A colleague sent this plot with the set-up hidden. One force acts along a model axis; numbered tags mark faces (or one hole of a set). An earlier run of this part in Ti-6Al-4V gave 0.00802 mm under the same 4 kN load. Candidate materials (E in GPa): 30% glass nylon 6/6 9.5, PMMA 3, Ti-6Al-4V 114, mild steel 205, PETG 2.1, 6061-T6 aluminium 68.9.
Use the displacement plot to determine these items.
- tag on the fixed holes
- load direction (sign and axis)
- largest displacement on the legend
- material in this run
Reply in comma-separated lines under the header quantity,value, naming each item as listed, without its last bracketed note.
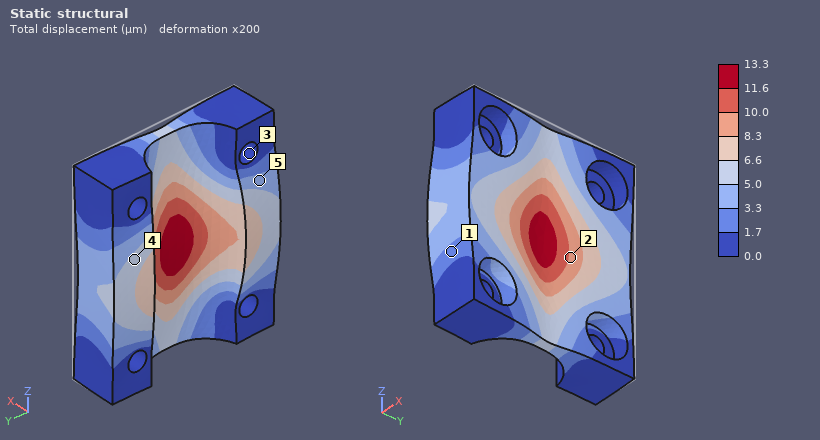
quantity,value
tag on the fixed holes,3
load direction,-X
largest displacement on the legend,13.3 µm
material in this run,6061-T6 aluminium
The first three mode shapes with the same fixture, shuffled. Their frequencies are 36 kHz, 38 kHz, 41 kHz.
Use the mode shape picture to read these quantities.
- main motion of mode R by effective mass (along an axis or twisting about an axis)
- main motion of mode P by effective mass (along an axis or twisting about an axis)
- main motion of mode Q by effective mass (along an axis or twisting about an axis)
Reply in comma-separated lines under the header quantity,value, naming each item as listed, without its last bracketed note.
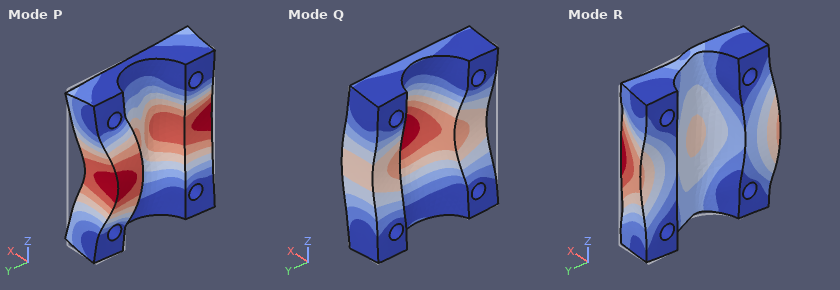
quantity,value
main motion of mode R by effective mass,along Y
main motion of mode P by effective mass,along Y
main motion of mode Q by effective mass,along X
